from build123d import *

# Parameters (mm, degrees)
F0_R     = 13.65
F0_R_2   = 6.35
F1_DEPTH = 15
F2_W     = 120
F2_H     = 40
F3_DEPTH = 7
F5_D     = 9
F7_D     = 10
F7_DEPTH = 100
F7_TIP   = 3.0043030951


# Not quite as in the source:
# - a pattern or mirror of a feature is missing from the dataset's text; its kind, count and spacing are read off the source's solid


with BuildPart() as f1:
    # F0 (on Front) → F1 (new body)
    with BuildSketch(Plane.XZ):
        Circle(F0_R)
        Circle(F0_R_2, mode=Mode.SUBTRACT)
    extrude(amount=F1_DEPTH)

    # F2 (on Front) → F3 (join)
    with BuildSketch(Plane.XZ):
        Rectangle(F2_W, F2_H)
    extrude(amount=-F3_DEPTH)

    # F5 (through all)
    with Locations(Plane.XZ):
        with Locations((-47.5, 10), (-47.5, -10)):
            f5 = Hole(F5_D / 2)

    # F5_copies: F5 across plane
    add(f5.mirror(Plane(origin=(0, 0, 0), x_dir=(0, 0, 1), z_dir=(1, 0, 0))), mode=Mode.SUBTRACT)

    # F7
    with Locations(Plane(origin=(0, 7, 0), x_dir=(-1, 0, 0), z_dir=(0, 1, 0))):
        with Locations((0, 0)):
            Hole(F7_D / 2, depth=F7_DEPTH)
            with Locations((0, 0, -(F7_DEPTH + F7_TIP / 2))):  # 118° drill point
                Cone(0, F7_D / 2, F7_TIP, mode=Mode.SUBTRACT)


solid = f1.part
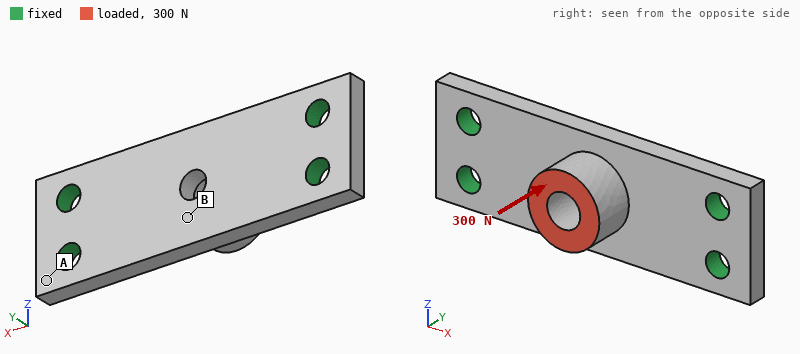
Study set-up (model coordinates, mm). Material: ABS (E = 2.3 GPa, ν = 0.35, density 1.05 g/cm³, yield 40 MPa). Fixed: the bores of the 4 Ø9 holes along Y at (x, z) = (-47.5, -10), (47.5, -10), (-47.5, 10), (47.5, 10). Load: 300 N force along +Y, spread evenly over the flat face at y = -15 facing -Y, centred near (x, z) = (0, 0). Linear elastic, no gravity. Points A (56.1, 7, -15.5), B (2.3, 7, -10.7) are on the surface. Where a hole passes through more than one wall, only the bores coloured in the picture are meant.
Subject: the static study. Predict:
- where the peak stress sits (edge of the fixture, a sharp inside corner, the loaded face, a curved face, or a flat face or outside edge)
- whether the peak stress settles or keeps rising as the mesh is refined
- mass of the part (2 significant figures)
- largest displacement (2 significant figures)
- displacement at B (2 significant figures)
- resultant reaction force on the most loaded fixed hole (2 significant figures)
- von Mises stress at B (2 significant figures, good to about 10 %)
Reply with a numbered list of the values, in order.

1. edge of the fixture
2. keeps rising
3. 40 g
4. 0.29 mm
5. 0.28 mm
6. 82 N
7. 3.2 MPa
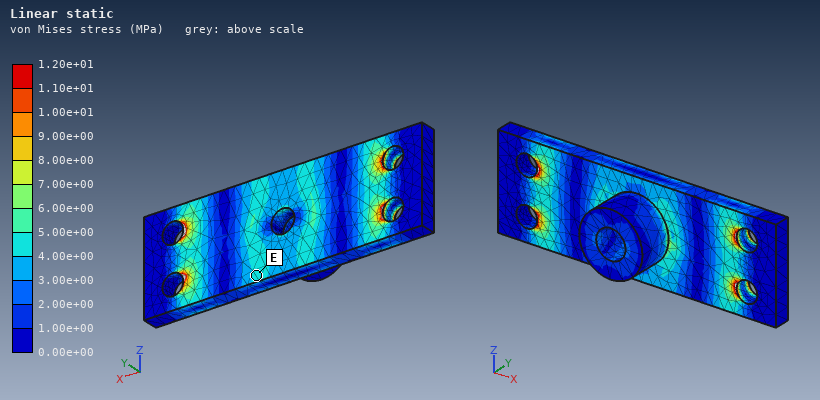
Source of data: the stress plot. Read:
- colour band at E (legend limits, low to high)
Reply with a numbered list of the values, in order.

1. 4.00e+00 to 5.00e+00 MPa
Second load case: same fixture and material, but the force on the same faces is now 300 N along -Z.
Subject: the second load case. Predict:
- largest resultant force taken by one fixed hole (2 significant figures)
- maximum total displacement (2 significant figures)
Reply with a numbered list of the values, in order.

1. 180 N
2. 0.49 mm
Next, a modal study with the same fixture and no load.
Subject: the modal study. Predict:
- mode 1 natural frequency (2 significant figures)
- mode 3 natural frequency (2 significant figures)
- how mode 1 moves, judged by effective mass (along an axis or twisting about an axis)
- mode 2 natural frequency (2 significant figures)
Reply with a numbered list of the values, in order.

1. 1200 Hz
2. 2800 Hz
3. along Y
4. 1600 Hz
